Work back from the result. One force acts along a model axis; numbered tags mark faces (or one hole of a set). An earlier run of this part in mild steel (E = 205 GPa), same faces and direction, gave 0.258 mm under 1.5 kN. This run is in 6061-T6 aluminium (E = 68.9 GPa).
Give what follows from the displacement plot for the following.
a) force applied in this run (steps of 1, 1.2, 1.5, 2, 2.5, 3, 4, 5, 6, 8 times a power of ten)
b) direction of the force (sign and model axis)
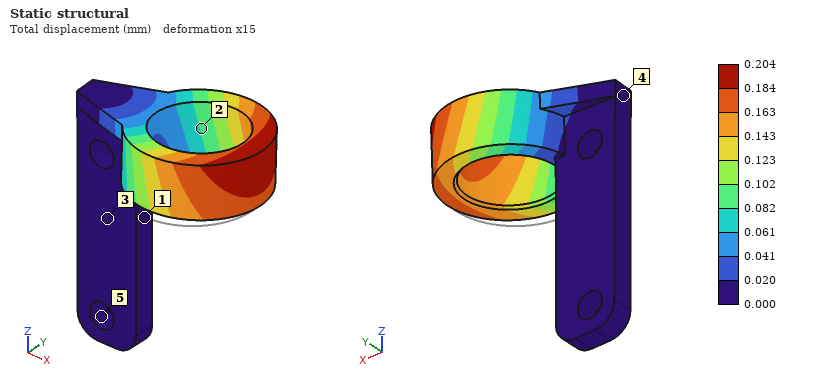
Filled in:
400 N
+Y
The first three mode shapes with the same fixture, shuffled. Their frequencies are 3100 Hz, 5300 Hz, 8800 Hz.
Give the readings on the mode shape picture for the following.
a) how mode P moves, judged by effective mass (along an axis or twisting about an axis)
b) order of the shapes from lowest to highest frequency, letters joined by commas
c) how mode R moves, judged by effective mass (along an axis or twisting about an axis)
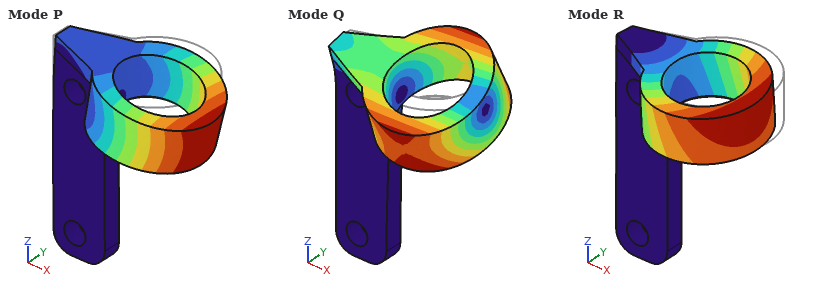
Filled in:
along Z
R, P, Q
along Y
